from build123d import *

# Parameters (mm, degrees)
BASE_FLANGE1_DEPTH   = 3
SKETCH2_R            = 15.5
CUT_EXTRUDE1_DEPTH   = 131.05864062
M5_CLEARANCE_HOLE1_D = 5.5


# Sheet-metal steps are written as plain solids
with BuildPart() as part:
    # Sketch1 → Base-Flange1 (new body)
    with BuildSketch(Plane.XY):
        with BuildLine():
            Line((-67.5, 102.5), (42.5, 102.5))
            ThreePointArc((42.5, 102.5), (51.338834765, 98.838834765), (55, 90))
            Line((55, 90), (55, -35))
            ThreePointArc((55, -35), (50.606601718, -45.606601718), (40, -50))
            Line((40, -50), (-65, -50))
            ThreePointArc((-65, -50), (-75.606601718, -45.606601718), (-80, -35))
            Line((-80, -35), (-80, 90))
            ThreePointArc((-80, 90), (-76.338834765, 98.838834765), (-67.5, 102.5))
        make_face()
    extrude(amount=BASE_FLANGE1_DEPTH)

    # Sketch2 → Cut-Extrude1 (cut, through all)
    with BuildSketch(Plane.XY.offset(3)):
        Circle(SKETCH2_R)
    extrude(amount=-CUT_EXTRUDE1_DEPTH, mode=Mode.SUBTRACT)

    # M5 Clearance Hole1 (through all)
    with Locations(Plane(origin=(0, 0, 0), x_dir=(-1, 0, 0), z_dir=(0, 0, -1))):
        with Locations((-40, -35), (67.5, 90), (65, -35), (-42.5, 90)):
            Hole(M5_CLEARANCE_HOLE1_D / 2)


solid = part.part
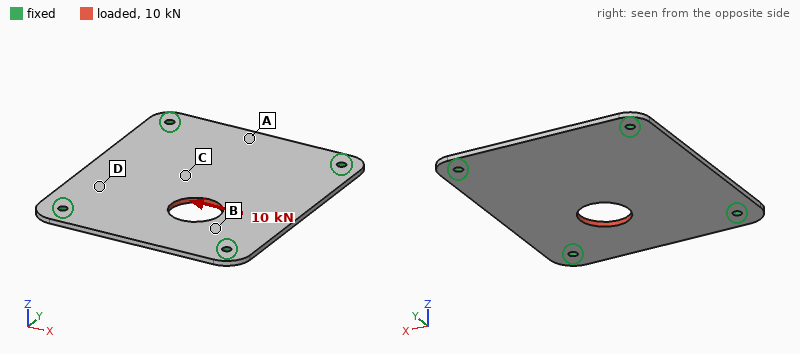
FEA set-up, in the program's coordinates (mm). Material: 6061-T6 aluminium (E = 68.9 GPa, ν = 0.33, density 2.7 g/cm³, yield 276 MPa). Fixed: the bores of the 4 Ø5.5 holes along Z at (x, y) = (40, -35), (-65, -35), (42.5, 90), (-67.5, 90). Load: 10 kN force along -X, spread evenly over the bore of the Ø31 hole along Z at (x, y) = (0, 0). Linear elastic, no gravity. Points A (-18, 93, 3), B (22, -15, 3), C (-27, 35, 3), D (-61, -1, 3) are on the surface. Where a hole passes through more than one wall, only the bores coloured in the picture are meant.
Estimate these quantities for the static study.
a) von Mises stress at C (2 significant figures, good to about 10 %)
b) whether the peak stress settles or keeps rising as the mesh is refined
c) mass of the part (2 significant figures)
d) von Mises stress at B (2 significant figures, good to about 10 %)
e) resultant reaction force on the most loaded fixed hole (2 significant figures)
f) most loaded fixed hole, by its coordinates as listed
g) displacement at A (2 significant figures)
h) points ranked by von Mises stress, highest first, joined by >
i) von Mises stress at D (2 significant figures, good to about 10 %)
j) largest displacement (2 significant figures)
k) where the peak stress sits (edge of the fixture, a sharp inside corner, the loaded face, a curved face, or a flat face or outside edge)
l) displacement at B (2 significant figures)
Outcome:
19 MPa
keeps rising
160 g
37 MPa
3.8 kN
(40, -35)
7.9 µm
B > C > D > A
11 MPa
47 µm
edge of the fixture
28 µm
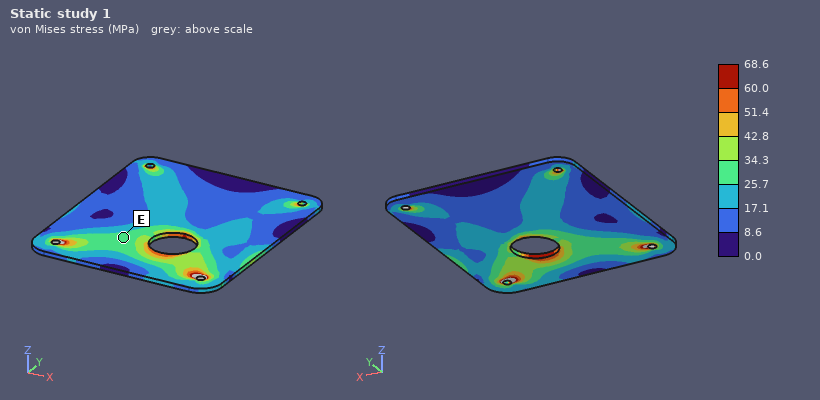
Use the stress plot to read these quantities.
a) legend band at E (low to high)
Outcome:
25.7 to 34.3 MPa
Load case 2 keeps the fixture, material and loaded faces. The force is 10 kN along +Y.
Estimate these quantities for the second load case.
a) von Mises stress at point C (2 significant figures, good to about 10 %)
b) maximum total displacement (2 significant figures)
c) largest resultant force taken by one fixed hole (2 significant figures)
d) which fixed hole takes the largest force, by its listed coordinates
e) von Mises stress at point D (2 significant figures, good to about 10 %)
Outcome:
22 MPa
48 µm
3.7 kN
(40, -35)
13 MPa
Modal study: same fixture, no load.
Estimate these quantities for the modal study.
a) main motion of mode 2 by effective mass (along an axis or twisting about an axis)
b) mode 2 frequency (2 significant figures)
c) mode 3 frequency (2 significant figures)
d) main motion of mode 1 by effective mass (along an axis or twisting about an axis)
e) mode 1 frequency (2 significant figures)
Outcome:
twisting about Y
1100 Hz
1400 Hz
along Z
760 Hz
